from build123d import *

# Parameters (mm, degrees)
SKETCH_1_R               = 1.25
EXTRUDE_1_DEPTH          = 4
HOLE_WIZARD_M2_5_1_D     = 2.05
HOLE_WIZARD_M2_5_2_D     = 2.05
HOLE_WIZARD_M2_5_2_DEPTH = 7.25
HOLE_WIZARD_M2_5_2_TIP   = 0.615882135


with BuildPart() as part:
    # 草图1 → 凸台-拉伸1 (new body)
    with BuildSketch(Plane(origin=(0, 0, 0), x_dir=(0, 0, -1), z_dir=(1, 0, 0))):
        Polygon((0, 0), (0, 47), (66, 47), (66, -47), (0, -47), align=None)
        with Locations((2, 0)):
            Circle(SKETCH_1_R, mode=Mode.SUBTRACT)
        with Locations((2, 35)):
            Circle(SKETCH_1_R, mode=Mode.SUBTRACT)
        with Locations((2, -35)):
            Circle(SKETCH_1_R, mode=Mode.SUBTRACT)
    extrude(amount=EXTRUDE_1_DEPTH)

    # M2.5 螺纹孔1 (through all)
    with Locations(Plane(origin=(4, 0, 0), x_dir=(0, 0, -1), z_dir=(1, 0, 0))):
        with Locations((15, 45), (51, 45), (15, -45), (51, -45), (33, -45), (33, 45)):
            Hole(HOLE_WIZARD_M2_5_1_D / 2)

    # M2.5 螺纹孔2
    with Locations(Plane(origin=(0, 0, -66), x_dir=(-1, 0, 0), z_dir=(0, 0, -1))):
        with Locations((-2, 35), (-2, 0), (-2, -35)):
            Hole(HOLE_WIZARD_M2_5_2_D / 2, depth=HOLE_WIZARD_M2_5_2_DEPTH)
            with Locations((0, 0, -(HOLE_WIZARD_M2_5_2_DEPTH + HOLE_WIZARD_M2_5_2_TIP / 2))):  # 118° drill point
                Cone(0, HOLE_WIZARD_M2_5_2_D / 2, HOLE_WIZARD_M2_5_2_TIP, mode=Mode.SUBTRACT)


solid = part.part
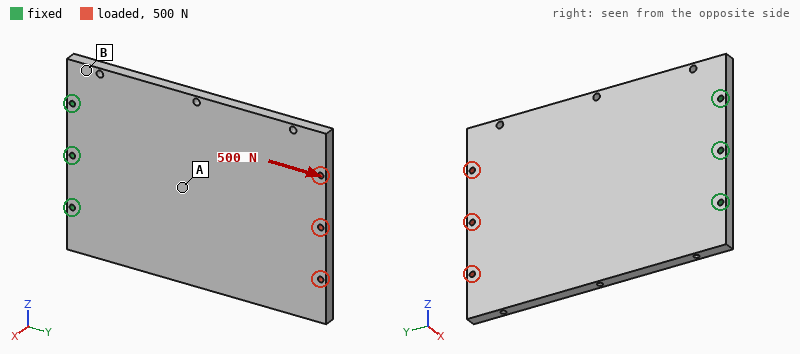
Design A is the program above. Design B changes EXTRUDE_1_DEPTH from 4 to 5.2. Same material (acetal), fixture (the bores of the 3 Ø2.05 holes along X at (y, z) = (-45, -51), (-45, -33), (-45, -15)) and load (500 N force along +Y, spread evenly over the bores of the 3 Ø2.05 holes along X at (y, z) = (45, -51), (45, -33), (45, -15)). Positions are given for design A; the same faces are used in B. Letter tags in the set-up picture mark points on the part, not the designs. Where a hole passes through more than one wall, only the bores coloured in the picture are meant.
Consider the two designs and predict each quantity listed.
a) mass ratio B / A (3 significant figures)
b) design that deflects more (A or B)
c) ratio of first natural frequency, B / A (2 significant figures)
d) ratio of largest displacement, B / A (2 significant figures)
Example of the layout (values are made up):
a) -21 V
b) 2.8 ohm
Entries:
a) 1.30
b) A
c) 1.3
d) 0.77
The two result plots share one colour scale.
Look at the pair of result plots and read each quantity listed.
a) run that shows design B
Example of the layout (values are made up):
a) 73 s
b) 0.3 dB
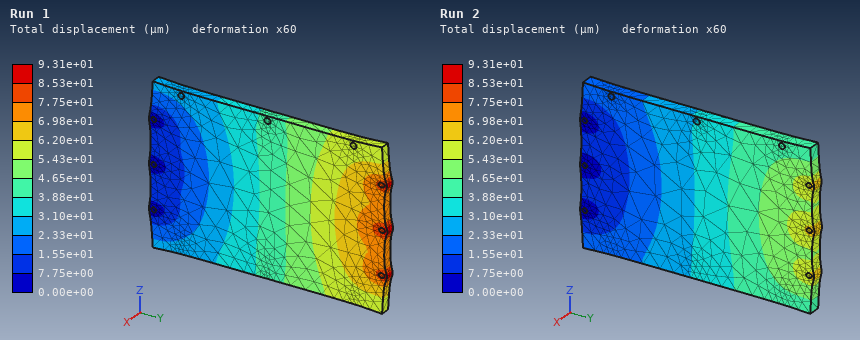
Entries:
a) Run 2
